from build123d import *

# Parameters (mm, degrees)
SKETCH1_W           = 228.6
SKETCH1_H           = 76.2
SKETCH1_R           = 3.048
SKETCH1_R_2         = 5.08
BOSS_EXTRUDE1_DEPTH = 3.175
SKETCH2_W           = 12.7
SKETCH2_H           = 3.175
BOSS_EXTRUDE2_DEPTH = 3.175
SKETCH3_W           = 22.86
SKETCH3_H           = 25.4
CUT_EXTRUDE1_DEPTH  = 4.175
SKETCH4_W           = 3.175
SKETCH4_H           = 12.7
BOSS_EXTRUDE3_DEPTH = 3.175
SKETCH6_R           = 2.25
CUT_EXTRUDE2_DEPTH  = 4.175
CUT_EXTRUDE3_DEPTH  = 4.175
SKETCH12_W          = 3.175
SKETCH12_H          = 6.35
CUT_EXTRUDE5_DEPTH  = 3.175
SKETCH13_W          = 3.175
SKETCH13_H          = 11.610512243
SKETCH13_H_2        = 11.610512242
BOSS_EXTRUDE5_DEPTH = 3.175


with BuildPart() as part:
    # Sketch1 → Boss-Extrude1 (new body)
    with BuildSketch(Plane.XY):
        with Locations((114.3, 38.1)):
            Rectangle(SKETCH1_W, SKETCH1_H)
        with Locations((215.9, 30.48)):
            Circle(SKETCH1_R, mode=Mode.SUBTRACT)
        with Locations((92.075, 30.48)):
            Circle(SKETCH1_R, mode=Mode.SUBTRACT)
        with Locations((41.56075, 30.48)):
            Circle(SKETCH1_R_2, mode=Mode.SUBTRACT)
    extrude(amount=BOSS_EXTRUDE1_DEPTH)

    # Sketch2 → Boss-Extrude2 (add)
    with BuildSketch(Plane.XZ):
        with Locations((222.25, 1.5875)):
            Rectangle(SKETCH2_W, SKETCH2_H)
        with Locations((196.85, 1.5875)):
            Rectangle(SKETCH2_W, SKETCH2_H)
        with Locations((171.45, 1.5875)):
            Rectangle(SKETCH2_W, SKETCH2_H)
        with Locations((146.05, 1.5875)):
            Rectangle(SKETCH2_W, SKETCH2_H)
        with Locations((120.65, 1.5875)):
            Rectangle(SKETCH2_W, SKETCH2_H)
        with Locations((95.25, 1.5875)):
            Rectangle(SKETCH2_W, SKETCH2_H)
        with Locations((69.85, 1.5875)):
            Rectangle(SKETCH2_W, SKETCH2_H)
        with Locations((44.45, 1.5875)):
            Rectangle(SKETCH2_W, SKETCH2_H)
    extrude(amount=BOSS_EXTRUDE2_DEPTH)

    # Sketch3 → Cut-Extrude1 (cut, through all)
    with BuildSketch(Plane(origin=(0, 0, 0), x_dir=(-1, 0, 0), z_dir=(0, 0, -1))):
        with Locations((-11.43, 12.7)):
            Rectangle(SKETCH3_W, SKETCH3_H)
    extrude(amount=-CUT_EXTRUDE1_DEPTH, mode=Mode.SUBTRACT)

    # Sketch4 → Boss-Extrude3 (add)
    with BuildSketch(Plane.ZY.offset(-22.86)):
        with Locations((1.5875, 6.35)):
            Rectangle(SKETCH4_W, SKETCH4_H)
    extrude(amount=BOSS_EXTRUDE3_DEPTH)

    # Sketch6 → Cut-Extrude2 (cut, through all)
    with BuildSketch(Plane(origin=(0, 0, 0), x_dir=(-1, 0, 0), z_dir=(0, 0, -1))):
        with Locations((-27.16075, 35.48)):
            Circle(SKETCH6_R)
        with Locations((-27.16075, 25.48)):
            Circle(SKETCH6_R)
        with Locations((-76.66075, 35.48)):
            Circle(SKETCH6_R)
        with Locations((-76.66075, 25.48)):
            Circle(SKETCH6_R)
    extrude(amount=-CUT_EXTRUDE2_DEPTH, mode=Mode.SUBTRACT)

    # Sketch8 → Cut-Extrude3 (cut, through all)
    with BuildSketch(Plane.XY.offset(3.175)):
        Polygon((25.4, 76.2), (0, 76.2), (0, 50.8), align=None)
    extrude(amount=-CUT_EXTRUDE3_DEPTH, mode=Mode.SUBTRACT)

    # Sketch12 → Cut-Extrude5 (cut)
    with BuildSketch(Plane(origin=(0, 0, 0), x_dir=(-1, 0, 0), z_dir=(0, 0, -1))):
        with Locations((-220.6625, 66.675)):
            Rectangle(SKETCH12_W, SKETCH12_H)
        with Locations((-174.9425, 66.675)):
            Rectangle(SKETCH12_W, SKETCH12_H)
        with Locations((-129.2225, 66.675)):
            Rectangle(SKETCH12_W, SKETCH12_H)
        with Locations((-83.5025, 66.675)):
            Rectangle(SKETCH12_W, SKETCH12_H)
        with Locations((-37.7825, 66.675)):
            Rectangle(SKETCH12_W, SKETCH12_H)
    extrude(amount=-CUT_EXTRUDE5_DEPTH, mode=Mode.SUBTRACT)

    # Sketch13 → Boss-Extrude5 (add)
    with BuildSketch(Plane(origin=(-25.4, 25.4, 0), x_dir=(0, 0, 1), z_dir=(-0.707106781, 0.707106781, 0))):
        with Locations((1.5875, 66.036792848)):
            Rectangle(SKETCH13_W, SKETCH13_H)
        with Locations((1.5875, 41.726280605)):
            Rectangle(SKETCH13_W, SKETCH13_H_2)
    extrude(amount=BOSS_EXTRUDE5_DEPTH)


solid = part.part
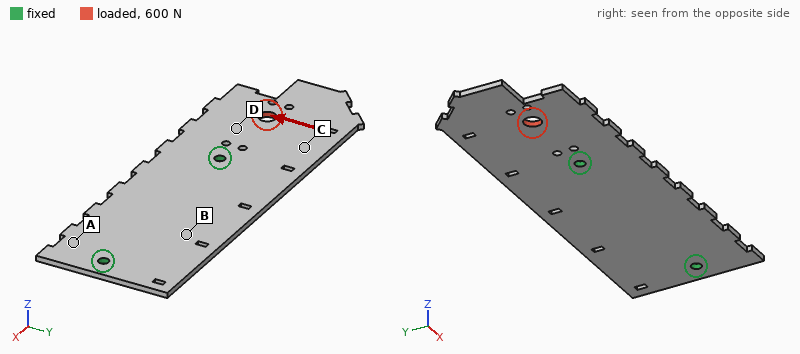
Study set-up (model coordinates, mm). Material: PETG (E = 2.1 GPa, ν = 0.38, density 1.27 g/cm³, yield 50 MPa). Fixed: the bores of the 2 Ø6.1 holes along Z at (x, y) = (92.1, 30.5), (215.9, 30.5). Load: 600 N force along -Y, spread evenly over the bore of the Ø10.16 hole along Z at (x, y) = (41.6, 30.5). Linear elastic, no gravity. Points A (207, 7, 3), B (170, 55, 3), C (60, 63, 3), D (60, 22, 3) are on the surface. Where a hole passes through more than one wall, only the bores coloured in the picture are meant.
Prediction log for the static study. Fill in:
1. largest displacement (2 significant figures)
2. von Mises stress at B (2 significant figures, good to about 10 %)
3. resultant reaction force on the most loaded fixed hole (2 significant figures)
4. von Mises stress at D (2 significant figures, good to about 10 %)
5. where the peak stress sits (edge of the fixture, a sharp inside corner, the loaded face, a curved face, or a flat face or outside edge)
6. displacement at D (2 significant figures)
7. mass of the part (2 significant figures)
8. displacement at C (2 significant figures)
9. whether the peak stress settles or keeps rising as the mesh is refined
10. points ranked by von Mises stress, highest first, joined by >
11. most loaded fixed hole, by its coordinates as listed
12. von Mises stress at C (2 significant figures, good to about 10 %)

1.1 mm
2.8 MPa
840 N
5.5 MPa
edge of the fixture
0.44 mm
67 g
0.51 mm
keeps rising
D > C > B > A
(92.1, 30.5)
4.3 MPa
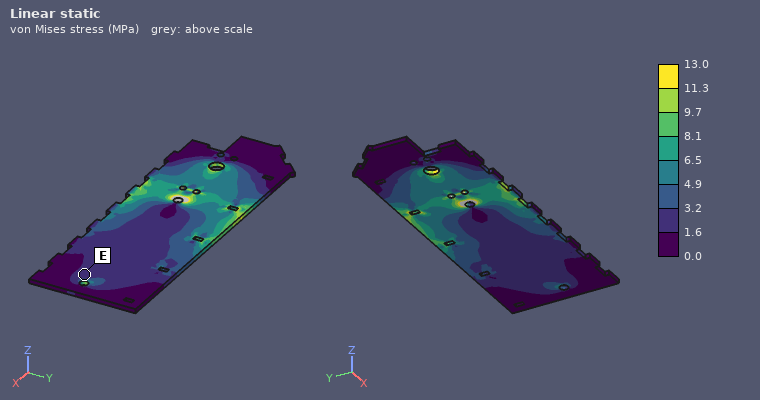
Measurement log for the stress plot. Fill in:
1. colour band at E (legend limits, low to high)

1.6 to 3.2 MPa
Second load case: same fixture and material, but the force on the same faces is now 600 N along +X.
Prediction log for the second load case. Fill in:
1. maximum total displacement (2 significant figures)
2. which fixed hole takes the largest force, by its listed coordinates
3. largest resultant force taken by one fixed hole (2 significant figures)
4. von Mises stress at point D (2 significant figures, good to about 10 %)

0.19 mm
(92.1, 30.5)
500 N
4.8 MPa
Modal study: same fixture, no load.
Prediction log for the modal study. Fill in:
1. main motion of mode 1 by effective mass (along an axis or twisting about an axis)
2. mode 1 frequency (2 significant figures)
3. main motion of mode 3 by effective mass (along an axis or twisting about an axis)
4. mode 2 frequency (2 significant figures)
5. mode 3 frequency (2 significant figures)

along Z
86 Hz
along Z
180 Hz
220 Hz
